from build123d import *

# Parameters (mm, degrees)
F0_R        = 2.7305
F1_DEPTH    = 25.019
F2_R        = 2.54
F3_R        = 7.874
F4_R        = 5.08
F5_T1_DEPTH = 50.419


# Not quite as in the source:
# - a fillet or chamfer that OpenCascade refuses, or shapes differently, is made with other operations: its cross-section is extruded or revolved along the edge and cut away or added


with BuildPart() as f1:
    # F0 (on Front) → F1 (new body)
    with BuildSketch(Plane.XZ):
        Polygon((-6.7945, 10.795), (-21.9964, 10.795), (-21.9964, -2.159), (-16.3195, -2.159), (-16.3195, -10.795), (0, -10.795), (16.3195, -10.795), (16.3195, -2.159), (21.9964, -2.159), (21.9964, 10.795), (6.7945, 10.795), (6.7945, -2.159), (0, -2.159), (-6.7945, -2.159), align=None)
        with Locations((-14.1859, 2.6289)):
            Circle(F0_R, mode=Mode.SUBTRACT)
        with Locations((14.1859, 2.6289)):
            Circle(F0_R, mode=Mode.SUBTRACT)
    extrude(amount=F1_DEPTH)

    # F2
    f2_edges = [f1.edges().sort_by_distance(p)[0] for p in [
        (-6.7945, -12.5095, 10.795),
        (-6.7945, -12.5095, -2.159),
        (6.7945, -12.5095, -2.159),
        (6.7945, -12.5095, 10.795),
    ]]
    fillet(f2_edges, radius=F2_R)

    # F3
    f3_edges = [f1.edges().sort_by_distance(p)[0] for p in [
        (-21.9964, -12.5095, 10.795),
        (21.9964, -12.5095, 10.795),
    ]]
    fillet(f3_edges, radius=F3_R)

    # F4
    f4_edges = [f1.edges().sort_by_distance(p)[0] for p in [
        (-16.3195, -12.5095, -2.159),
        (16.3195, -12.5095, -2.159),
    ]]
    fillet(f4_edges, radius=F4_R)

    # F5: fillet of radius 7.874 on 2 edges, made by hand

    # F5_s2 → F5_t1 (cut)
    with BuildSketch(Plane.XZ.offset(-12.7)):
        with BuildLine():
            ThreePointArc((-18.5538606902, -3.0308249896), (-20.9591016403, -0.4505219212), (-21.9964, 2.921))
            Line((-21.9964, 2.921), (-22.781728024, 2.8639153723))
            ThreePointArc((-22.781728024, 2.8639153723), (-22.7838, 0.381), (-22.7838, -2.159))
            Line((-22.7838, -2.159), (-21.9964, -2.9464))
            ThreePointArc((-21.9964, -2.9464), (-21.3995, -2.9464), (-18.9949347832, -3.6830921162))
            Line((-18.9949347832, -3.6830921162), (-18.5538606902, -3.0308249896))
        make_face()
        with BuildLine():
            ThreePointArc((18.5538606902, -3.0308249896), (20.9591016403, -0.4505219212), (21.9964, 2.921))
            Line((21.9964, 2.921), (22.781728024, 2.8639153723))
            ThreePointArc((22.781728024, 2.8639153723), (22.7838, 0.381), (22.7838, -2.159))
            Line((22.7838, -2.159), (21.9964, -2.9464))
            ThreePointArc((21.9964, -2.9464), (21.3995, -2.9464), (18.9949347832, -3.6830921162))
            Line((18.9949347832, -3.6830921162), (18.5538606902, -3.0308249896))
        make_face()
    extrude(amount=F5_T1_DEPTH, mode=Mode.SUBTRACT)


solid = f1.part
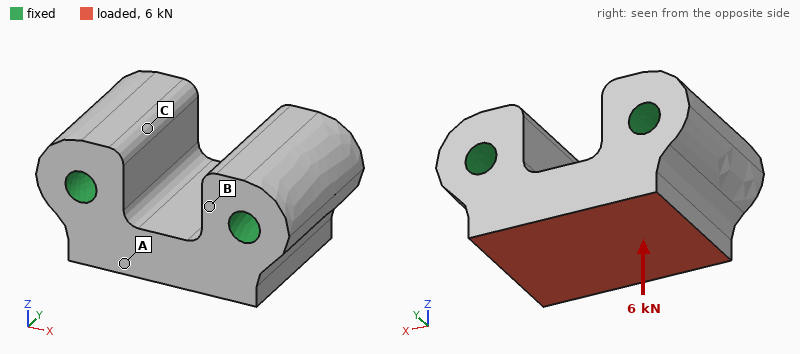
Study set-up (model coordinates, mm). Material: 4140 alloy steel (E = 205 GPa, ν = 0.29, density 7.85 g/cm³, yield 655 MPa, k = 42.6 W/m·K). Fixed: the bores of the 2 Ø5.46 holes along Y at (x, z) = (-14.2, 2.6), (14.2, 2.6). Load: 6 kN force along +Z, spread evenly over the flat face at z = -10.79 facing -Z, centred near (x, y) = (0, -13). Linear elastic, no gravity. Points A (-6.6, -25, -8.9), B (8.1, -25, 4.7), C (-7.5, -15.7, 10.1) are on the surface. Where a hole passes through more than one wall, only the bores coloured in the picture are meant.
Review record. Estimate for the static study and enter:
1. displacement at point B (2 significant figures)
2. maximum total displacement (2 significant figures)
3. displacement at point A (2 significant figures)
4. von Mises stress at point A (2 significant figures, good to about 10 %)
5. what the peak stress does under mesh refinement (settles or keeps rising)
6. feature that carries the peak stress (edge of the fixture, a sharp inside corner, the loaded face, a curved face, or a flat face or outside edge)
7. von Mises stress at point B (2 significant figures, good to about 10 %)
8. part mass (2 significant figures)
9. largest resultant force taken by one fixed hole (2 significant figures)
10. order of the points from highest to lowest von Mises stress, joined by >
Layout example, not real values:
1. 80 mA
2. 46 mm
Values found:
1. 0.29 µm
2. 1.4 µm
3. 0.98 µm
4. 8.9 MPa
5. keeps rising
6. edge of the fixture
7. 5.3 MPa
8. 120 g
9. 3.2 kN
10. A > B > C
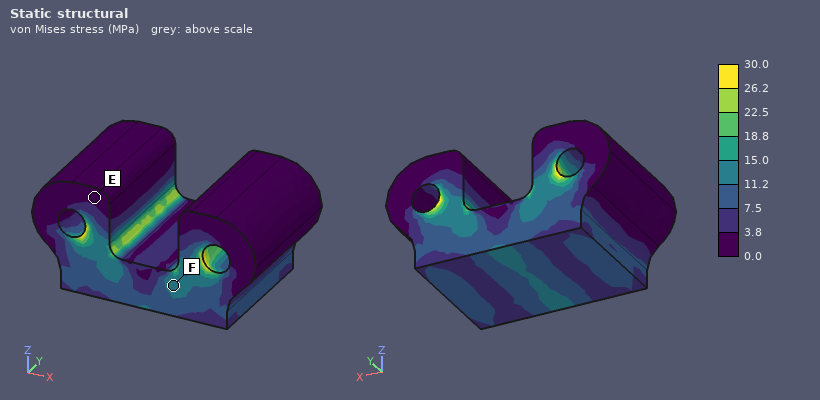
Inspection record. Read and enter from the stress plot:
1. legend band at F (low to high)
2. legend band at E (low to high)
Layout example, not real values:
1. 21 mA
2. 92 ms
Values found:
1. 11.2 to 15.0 MPa
2. 0.0 to 3.8 MPa
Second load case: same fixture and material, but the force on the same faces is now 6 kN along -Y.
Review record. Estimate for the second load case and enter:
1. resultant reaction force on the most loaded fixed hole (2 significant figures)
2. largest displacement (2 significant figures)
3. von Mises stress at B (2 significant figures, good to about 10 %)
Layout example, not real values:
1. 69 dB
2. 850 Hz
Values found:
1. 3.0 kN
2. 3.8 µm
3. 13 MPa
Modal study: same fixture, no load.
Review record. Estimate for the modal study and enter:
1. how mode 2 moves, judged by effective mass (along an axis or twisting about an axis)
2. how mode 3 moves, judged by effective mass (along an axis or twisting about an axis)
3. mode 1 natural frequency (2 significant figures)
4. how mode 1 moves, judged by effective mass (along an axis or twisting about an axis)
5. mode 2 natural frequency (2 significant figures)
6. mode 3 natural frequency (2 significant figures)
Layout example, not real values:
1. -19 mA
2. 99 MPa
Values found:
1. along X
2. along Z
3. 41 kHz
4. along Y
5. 45 kHz
6. 51 kHz
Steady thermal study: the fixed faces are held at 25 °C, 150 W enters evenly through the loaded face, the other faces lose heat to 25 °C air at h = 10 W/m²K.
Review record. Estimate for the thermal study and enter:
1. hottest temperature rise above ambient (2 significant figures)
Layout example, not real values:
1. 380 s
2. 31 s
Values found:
1. 79 K
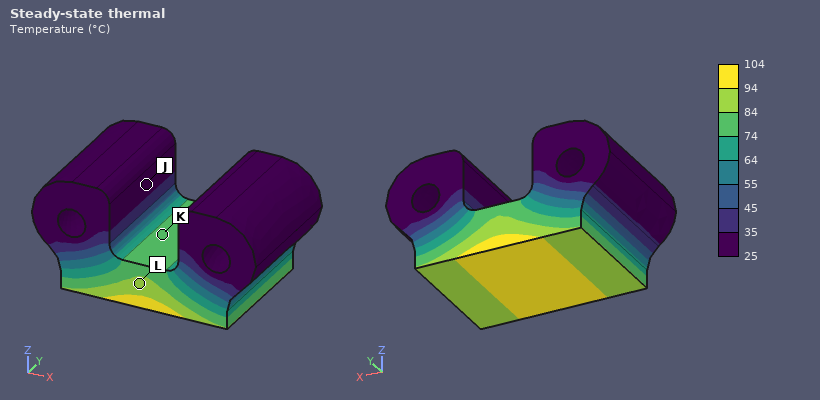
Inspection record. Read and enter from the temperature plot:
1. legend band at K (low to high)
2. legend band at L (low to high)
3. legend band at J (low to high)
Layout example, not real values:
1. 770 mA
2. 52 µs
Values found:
1. 74 to 84 °C
2. 84 to 94 °C
3. 25 to 35 °C
